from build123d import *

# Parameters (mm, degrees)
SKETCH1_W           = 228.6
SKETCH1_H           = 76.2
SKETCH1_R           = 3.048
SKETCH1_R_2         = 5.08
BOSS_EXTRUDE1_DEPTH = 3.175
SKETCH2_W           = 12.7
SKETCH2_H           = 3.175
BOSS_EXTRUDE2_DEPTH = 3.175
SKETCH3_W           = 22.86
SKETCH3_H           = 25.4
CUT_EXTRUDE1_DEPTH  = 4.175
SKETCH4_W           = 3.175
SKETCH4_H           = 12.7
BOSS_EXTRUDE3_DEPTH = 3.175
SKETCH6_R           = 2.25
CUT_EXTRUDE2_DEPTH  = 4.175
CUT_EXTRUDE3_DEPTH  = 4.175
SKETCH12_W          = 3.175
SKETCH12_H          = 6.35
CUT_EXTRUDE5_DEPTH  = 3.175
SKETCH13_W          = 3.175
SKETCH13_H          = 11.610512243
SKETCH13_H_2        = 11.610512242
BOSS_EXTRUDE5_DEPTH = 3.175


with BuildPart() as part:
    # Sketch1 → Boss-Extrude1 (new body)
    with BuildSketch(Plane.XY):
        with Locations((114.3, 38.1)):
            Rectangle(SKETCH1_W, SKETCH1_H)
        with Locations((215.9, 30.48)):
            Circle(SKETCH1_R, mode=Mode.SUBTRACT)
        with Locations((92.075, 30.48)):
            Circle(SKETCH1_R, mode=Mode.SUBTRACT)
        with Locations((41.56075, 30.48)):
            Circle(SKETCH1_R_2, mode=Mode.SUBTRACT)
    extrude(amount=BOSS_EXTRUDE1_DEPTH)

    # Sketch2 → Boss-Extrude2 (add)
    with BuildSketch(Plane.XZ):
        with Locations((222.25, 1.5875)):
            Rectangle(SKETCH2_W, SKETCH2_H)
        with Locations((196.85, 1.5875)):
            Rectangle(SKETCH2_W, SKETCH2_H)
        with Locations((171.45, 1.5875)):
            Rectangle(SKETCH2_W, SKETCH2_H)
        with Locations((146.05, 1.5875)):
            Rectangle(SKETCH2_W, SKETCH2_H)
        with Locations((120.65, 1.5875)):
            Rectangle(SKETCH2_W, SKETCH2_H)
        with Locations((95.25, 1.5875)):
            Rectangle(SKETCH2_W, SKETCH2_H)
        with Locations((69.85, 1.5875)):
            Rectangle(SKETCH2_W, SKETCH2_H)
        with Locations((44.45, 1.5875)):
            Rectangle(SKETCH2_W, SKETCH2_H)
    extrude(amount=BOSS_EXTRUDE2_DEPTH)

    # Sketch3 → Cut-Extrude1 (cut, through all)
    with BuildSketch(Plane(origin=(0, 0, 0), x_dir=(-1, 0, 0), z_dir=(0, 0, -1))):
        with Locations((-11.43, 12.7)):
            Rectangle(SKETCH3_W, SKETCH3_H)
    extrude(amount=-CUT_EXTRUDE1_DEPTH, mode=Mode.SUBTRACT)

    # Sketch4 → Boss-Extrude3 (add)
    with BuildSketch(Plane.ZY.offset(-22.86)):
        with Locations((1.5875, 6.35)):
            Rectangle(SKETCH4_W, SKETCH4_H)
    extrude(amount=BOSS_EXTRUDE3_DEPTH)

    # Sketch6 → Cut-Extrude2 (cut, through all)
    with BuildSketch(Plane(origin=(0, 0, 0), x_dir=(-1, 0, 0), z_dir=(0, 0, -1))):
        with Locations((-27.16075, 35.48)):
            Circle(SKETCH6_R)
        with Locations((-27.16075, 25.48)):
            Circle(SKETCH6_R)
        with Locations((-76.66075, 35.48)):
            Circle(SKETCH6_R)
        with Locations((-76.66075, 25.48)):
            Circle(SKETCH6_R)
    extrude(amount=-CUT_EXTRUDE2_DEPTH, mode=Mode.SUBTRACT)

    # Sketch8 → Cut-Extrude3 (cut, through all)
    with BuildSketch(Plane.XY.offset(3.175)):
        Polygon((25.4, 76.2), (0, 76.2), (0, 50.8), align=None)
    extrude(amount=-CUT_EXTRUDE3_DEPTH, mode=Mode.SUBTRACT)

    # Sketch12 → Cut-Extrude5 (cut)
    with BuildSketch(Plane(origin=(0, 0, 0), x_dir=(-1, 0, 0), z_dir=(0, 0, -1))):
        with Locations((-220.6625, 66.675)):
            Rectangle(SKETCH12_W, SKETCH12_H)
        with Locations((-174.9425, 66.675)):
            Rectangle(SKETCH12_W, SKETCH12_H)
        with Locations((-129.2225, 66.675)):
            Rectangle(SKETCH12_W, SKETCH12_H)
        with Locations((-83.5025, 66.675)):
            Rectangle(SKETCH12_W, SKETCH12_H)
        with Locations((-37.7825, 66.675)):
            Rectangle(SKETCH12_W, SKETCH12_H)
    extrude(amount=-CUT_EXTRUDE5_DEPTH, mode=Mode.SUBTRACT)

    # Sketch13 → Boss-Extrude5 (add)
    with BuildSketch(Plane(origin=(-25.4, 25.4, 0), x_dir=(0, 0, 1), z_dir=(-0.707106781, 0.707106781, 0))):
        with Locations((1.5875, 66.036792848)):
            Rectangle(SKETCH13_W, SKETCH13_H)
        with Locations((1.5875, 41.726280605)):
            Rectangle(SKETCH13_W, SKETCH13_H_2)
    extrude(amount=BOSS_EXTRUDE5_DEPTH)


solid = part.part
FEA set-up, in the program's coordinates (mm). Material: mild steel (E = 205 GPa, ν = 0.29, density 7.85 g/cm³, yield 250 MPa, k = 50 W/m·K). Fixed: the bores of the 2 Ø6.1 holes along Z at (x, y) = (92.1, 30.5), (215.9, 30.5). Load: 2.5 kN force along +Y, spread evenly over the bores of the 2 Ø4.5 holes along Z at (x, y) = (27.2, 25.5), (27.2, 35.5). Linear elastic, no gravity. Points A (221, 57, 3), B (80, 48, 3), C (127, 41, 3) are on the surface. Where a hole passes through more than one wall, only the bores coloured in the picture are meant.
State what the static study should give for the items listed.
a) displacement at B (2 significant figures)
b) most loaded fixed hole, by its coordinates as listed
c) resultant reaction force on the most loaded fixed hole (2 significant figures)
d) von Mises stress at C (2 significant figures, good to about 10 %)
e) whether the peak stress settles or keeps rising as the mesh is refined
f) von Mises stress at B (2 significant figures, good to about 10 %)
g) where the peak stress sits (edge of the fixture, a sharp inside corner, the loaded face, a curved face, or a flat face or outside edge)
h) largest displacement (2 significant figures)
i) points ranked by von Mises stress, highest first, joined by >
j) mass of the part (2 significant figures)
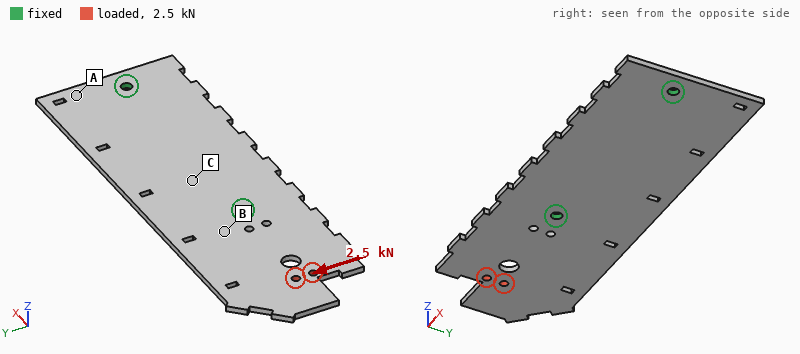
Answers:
10 µm
(92.1, 30.5)
3.8 kN
13 MPa
keeps rising
32 MPa
edge of the fixture
64 µm
B > C > A
410 g
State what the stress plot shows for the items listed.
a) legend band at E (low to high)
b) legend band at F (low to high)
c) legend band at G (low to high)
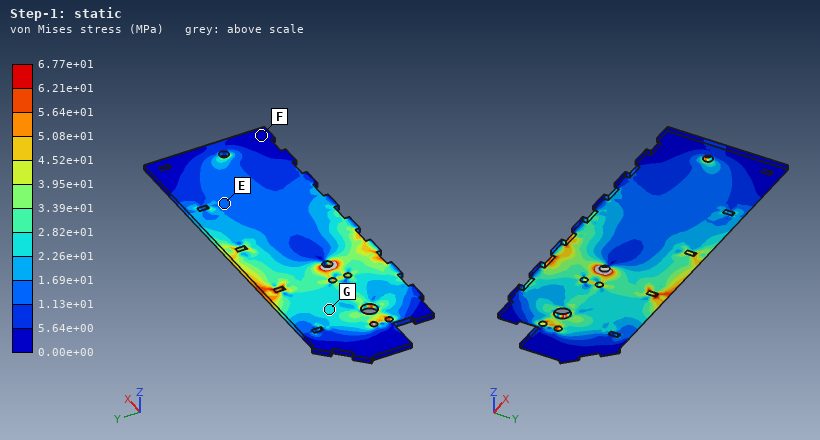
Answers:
1.13e+01 to 1.69e+01 MPa
0.00e+00 to 5.64e+00 MPa
2.26e+01 to 2.82e+01 MPa
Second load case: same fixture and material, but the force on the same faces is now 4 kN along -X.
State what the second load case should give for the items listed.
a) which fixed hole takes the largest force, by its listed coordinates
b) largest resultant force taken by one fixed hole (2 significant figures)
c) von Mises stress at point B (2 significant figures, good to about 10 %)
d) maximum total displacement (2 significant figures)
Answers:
(92.1, 30.5)
3.3 kN
14 MPa
20 µm
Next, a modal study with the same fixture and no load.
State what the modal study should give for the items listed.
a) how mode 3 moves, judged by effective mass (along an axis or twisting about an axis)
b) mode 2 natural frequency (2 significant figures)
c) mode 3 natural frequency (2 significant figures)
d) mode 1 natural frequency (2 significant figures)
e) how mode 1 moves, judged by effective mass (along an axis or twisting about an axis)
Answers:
along Z
720 Hz
860 Hz
340 Hz
along Z
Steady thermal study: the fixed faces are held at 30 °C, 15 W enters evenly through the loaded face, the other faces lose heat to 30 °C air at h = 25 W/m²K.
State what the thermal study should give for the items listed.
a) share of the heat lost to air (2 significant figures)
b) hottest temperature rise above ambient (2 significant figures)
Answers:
72 %
73 K
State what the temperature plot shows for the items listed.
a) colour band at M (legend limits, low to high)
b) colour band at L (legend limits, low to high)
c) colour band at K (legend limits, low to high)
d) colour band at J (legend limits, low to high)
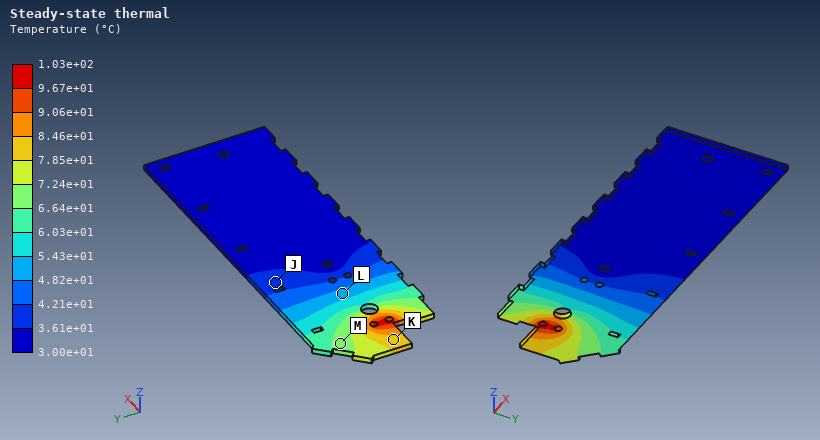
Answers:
6.64e+01 to 7.24e+01 °C
4.82e+01 to 5.43e+01 °C
7.85e+01 to 8.46e+01 °C
3.61e+01 to 4.21e+01 °C
